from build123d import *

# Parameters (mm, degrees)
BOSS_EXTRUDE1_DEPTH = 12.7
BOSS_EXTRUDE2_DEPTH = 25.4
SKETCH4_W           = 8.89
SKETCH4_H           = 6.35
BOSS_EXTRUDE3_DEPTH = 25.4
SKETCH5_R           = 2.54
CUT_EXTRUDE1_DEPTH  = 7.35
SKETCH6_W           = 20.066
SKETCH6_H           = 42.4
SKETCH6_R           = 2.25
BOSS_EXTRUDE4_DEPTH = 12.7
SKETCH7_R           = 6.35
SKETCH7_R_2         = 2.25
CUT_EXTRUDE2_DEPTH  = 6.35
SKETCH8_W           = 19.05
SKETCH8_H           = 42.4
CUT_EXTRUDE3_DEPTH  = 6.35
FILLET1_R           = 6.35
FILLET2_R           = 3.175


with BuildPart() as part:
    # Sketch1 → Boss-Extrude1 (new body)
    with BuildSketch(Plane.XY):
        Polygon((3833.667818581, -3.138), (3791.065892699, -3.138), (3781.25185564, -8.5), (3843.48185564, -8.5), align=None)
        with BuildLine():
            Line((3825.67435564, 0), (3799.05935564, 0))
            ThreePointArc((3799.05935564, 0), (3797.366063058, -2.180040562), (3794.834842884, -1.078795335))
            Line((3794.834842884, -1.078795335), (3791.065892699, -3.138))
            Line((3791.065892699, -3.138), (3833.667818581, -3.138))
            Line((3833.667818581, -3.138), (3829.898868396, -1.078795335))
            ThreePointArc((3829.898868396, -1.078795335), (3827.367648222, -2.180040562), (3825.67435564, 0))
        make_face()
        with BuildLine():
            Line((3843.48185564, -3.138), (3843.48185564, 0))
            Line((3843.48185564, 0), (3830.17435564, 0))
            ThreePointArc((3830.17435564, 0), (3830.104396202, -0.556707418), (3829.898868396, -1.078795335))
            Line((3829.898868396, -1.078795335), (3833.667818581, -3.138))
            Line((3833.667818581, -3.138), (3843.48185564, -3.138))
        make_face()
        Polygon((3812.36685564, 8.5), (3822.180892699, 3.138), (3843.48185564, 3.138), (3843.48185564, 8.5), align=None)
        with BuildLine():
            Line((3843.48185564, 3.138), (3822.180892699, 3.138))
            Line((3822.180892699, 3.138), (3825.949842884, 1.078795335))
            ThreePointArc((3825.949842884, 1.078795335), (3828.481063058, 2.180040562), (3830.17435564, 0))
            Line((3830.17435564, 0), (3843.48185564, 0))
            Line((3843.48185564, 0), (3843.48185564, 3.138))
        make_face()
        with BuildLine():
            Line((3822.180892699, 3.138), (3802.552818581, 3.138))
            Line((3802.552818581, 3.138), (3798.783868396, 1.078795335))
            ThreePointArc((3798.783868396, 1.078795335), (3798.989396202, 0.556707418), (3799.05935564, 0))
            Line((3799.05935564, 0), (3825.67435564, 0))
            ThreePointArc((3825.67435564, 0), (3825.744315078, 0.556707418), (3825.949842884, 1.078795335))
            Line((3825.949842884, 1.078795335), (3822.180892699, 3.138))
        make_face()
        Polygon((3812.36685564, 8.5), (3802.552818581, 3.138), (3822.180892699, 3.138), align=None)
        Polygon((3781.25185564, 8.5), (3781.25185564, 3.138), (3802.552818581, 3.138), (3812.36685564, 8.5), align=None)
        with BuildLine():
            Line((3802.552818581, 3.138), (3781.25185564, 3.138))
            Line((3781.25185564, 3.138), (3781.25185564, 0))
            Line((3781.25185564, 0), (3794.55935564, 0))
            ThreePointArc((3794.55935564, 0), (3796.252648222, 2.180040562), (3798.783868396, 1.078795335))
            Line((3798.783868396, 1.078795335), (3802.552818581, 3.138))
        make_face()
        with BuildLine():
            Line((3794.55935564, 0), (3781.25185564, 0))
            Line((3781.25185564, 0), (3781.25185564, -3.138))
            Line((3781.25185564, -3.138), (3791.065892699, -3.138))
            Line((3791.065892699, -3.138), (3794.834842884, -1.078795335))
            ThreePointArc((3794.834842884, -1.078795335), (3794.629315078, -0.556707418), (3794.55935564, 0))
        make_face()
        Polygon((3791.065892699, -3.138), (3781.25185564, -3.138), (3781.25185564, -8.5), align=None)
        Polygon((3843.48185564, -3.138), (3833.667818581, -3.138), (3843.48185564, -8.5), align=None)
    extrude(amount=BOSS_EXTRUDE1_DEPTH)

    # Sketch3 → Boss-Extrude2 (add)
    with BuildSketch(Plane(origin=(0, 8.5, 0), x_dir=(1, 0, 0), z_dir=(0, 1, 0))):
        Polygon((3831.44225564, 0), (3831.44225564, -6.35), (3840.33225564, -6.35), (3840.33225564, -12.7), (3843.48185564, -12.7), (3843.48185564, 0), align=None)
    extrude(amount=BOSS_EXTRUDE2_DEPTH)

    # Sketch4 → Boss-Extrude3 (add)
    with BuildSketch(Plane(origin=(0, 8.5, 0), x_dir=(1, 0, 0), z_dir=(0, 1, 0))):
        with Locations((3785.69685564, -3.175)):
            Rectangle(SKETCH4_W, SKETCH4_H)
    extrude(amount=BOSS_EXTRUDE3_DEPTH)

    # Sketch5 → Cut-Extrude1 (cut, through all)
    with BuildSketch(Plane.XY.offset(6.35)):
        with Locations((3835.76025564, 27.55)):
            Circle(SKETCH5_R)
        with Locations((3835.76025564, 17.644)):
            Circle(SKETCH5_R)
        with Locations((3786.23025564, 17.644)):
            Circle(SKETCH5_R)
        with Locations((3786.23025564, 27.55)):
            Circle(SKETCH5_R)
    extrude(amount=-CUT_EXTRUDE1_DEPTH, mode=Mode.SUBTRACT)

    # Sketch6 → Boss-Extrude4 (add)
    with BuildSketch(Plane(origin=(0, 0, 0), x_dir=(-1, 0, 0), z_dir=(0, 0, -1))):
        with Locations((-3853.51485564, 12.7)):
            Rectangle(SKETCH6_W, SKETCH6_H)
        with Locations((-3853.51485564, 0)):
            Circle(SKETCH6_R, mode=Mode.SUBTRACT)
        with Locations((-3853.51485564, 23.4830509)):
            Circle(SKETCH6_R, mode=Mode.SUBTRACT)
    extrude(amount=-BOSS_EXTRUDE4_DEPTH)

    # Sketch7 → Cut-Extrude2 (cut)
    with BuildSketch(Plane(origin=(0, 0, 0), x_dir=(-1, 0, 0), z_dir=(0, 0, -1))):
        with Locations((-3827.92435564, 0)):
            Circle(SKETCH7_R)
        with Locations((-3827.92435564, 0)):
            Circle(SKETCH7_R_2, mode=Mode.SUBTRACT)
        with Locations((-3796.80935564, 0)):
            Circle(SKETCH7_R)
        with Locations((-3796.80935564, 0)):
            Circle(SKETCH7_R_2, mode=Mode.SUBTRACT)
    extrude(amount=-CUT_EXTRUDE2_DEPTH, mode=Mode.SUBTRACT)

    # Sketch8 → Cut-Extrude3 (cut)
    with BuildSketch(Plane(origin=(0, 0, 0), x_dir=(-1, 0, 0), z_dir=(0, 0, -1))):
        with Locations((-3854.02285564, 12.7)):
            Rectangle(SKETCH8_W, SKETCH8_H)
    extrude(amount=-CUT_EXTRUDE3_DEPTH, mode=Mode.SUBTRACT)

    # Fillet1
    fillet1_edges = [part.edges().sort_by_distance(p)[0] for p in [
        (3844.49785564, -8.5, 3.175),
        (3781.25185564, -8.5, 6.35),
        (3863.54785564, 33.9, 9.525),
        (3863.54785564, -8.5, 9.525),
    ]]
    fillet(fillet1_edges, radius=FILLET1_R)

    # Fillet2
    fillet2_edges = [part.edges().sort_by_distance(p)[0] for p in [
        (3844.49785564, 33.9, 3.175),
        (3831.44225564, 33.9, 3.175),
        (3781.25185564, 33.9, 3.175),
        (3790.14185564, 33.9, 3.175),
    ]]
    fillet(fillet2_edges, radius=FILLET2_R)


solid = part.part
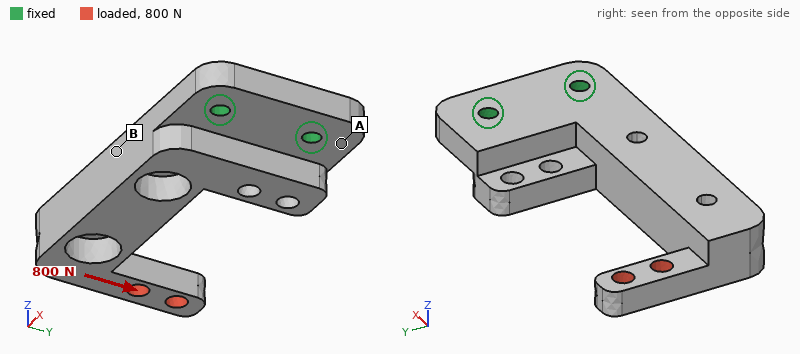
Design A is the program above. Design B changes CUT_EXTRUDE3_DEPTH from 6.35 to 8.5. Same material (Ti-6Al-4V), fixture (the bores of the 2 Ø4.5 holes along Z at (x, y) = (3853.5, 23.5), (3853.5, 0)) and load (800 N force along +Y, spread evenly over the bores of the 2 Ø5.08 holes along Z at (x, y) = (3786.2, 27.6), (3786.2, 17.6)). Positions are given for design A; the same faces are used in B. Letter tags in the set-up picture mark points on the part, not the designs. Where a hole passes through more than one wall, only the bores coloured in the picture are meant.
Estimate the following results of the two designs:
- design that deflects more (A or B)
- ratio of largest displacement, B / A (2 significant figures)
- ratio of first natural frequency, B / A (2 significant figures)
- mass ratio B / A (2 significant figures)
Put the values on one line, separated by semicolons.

B; 1.2; 0.66; 0.92
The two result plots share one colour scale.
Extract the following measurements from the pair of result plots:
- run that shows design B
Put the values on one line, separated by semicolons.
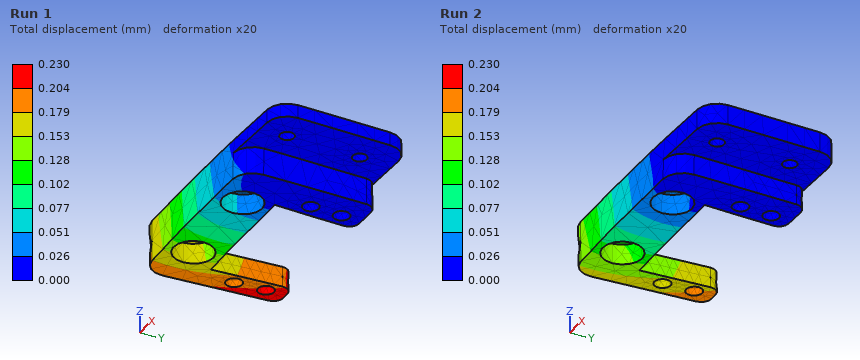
Run 1
